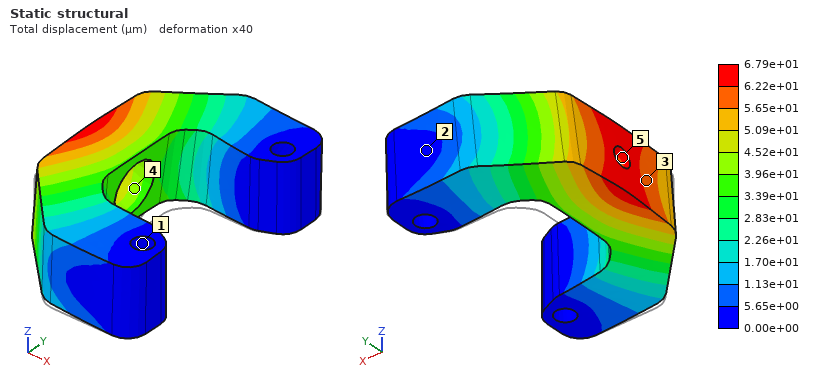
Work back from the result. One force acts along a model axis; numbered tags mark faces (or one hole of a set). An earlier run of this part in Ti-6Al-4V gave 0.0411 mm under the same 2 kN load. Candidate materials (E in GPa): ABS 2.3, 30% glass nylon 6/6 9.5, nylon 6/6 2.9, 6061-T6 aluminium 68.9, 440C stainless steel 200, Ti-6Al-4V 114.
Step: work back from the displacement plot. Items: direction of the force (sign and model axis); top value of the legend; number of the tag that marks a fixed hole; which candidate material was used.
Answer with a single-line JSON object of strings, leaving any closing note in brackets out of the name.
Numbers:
{"direction of the force": "+Z", "top value of the legend": "6.79e+01 µm", "number of the tag that marks a fixed hole": "1", "which candidate material was used": "6061-T6 aluminium"}
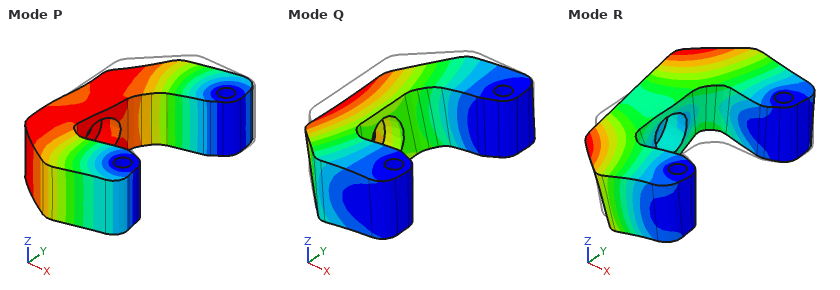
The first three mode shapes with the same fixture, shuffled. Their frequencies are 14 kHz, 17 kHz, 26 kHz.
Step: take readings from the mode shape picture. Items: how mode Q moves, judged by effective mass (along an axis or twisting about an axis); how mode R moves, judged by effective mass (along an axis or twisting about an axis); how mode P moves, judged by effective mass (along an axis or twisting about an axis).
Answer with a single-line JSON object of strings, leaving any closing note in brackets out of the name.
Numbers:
{"how mode Q moves, judged by effective mass": "along Z", "how mode R moves, judged by effective mass": "twisting about X", "how mode P moves, judged by effective mass": "along Y"}
